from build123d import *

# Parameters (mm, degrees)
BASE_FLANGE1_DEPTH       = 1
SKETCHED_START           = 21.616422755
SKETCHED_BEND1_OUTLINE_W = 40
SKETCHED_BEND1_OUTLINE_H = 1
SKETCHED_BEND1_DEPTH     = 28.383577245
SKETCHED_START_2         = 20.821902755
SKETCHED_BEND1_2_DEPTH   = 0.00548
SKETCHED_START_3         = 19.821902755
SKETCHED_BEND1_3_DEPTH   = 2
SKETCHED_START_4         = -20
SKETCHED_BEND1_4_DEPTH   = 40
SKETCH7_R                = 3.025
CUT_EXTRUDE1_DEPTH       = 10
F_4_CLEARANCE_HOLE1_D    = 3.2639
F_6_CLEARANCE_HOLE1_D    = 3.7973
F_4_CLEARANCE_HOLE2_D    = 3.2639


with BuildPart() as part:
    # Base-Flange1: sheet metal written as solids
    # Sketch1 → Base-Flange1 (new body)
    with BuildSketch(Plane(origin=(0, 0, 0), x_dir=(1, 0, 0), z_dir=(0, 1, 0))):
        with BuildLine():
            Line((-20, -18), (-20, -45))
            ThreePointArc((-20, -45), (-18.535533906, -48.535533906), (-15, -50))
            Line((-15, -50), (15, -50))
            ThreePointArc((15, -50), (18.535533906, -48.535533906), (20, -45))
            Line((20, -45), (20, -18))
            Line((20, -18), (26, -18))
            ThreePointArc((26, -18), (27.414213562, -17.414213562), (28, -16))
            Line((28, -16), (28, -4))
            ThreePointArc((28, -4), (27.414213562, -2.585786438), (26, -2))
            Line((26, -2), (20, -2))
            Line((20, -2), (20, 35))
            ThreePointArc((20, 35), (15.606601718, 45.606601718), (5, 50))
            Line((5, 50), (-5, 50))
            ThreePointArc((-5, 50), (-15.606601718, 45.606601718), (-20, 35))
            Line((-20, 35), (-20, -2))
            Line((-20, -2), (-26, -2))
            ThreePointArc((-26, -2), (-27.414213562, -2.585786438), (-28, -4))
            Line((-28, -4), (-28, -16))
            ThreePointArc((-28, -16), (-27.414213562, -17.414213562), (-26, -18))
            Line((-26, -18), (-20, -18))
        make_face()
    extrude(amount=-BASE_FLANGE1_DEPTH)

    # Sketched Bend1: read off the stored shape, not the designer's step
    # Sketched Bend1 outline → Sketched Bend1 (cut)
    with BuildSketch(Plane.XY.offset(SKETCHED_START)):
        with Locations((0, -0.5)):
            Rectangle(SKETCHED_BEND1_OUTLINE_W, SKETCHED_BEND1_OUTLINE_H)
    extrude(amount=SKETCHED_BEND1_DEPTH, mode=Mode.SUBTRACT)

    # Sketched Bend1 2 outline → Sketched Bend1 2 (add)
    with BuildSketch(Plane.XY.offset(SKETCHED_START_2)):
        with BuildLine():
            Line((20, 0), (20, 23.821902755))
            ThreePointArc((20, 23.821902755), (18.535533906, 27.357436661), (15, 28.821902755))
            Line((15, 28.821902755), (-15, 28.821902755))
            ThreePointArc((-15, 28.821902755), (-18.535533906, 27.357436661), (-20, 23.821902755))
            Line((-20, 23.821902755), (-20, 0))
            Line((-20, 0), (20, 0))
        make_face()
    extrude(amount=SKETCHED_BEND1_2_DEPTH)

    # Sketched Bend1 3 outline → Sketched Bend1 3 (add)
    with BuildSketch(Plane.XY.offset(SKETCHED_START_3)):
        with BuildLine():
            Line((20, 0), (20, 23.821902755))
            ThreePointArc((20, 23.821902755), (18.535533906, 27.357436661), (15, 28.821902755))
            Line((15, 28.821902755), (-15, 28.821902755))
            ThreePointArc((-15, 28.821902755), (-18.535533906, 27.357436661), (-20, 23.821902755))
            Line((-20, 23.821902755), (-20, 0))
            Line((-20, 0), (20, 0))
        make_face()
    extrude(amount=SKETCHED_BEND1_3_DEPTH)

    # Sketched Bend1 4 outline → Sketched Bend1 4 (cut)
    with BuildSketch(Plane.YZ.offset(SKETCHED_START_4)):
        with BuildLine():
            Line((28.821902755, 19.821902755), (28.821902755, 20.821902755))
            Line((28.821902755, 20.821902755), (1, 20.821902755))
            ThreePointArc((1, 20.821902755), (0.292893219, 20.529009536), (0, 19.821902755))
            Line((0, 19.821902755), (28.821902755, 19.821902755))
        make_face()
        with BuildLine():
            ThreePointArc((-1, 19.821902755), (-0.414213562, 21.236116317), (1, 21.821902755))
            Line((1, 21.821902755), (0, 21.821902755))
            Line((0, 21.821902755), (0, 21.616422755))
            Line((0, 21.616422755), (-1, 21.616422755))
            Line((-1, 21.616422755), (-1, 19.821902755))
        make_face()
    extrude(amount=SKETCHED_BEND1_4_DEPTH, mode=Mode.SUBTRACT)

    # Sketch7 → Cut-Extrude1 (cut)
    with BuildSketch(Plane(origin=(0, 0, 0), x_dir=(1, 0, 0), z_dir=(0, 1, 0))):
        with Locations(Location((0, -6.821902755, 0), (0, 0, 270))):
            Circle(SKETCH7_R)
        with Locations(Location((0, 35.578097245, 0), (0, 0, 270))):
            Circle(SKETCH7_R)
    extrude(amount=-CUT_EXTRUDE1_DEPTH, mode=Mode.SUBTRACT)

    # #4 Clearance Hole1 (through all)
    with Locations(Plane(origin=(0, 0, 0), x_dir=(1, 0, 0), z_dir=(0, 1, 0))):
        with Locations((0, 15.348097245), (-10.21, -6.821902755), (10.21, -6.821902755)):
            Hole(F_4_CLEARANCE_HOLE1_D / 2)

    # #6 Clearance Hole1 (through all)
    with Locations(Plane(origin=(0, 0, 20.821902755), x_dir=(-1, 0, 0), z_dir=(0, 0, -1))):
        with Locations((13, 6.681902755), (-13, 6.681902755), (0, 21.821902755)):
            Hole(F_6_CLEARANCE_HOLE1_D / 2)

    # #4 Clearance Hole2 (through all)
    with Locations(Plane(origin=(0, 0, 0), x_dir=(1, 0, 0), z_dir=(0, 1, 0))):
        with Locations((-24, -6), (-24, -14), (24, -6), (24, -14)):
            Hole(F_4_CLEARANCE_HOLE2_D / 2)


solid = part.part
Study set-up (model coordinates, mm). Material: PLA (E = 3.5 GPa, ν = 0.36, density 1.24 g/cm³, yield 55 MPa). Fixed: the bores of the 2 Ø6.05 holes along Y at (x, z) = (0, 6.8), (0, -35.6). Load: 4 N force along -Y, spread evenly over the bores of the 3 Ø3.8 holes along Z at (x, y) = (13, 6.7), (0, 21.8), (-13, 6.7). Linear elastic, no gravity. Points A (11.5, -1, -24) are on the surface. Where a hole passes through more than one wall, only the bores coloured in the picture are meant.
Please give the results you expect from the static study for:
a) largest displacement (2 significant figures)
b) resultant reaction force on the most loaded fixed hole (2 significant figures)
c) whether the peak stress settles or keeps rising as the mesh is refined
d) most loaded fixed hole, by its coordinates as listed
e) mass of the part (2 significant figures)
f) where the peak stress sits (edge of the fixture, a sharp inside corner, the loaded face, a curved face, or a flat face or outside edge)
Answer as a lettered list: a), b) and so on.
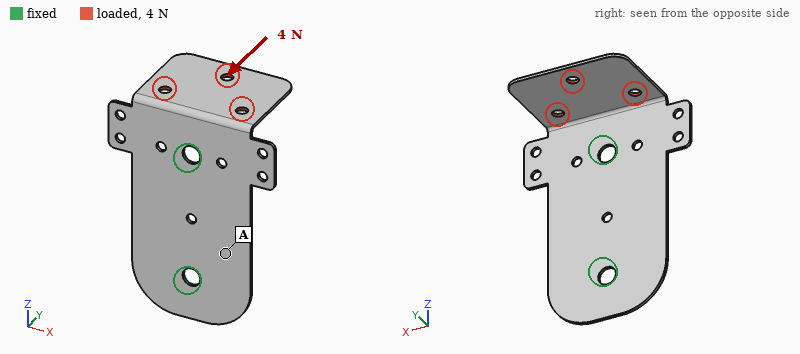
a) 0.96 mm
b) 4.2 N
c) keeps rising
d) (0, 6.8)
e) 5.0 g
f) edge of the fixture
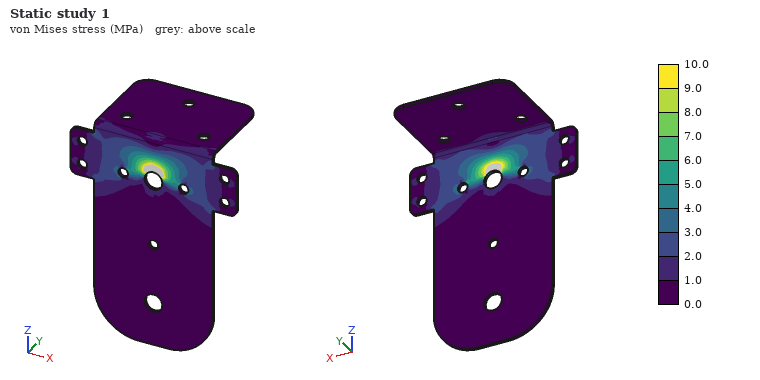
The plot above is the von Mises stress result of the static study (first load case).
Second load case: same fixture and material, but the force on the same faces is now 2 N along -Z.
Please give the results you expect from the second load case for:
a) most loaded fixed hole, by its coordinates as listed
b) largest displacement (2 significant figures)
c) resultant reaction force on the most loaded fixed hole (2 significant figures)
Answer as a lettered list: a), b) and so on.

a) (0, 6.8)
b) 1.1 mm
c) 1.6 N
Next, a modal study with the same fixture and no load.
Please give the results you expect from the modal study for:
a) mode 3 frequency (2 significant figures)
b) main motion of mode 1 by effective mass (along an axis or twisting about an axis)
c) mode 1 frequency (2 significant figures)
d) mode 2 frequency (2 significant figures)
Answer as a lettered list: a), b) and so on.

a) 540 Hz
b) along Z
c) 190 Hz
d) 250 Hz
